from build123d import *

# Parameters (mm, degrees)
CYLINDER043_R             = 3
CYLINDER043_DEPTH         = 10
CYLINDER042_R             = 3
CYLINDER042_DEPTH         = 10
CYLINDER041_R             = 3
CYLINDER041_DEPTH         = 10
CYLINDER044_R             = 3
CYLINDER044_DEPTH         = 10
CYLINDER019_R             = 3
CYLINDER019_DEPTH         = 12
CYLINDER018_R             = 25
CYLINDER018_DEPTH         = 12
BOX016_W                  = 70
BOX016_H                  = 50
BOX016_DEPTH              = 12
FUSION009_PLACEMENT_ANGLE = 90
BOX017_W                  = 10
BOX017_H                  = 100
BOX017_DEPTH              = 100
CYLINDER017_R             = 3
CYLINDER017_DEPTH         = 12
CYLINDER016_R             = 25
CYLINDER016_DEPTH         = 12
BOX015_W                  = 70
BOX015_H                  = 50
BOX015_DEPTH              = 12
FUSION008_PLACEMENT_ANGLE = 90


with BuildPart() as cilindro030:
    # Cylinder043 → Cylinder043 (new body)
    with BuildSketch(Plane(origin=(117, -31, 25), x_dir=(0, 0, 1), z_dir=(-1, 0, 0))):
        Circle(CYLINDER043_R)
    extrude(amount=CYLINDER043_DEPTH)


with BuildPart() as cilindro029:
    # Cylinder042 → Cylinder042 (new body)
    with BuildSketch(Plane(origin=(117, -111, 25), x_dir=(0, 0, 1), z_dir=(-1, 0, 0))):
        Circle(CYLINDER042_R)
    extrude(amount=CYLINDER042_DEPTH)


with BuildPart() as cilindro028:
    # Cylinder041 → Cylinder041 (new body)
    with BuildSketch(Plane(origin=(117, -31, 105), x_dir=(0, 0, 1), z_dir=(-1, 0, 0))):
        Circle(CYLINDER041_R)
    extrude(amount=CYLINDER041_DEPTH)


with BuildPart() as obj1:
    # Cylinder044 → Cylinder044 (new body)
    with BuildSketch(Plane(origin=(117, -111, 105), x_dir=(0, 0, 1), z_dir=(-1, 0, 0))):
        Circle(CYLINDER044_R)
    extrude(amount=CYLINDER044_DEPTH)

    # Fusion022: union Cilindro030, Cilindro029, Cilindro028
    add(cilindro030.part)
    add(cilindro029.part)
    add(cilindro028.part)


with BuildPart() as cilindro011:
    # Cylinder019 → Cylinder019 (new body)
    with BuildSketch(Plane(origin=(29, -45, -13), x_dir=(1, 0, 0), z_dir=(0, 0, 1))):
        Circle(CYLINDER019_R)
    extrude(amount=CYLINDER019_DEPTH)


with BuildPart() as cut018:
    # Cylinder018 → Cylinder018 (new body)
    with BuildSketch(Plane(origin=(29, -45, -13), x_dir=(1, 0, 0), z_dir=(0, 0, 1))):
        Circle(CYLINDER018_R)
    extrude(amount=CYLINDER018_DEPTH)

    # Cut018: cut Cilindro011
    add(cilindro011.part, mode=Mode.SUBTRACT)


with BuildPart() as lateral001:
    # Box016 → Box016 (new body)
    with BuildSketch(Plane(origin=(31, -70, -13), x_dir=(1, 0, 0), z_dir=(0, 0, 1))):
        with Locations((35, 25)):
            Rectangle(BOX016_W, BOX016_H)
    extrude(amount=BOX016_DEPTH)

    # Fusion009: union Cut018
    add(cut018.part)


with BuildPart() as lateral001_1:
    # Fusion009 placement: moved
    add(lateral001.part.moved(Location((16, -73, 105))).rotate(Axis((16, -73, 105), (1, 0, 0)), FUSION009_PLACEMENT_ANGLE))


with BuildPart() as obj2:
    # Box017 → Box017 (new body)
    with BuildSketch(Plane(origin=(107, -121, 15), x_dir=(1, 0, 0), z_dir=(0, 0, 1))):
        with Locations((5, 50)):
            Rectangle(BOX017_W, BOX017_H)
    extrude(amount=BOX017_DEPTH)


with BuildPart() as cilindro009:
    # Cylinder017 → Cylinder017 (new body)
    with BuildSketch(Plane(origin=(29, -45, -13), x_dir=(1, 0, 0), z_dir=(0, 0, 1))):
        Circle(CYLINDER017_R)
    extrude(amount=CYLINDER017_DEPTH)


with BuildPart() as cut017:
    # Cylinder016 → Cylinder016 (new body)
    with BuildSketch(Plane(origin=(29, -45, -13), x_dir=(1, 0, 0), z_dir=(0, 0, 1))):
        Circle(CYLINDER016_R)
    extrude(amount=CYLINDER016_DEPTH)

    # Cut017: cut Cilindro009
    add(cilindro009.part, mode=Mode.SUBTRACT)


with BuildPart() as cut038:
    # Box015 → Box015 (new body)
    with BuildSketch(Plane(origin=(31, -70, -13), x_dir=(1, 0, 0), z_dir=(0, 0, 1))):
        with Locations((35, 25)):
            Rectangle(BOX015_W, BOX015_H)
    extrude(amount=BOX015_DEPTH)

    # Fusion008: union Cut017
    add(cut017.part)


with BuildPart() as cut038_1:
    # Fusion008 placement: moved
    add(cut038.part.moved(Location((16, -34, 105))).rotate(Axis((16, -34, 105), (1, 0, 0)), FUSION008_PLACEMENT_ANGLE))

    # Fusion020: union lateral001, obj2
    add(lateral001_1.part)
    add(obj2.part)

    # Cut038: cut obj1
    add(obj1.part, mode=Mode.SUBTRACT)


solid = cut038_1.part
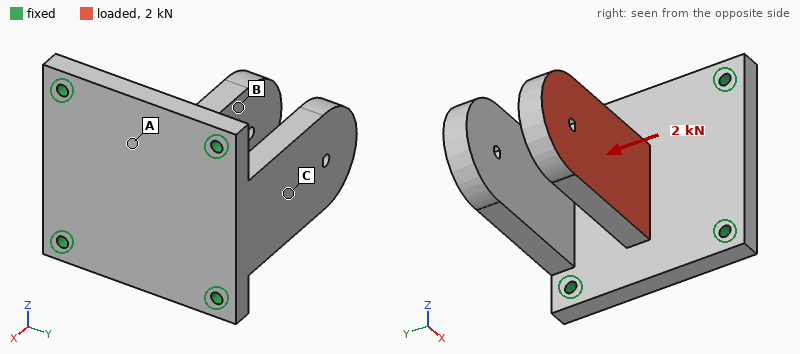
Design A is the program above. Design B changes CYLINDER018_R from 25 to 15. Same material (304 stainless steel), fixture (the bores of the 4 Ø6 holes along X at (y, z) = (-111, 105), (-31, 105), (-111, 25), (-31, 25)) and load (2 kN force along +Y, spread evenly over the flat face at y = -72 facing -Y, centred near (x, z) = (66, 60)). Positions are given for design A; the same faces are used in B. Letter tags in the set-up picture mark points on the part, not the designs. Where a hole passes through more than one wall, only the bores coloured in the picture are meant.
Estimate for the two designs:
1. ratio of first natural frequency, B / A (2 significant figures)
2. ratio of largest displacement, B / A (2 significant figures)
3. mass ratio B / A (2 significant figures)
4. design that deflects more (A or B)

1.0
0.68
0.96
A
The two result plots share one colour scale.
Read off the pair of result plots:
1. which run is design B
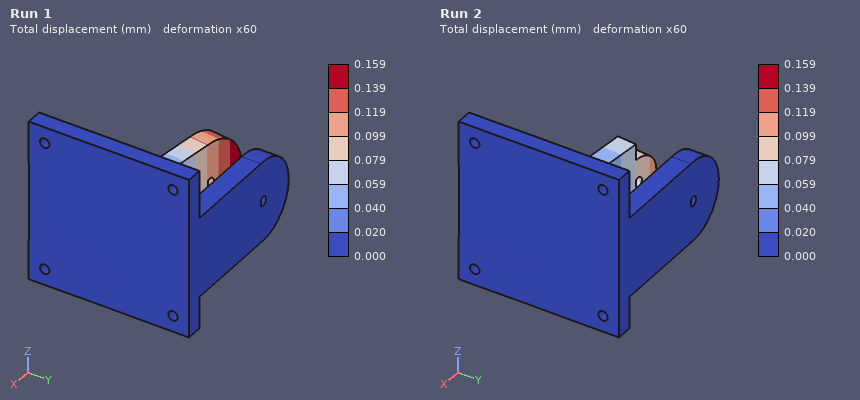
Run 2
